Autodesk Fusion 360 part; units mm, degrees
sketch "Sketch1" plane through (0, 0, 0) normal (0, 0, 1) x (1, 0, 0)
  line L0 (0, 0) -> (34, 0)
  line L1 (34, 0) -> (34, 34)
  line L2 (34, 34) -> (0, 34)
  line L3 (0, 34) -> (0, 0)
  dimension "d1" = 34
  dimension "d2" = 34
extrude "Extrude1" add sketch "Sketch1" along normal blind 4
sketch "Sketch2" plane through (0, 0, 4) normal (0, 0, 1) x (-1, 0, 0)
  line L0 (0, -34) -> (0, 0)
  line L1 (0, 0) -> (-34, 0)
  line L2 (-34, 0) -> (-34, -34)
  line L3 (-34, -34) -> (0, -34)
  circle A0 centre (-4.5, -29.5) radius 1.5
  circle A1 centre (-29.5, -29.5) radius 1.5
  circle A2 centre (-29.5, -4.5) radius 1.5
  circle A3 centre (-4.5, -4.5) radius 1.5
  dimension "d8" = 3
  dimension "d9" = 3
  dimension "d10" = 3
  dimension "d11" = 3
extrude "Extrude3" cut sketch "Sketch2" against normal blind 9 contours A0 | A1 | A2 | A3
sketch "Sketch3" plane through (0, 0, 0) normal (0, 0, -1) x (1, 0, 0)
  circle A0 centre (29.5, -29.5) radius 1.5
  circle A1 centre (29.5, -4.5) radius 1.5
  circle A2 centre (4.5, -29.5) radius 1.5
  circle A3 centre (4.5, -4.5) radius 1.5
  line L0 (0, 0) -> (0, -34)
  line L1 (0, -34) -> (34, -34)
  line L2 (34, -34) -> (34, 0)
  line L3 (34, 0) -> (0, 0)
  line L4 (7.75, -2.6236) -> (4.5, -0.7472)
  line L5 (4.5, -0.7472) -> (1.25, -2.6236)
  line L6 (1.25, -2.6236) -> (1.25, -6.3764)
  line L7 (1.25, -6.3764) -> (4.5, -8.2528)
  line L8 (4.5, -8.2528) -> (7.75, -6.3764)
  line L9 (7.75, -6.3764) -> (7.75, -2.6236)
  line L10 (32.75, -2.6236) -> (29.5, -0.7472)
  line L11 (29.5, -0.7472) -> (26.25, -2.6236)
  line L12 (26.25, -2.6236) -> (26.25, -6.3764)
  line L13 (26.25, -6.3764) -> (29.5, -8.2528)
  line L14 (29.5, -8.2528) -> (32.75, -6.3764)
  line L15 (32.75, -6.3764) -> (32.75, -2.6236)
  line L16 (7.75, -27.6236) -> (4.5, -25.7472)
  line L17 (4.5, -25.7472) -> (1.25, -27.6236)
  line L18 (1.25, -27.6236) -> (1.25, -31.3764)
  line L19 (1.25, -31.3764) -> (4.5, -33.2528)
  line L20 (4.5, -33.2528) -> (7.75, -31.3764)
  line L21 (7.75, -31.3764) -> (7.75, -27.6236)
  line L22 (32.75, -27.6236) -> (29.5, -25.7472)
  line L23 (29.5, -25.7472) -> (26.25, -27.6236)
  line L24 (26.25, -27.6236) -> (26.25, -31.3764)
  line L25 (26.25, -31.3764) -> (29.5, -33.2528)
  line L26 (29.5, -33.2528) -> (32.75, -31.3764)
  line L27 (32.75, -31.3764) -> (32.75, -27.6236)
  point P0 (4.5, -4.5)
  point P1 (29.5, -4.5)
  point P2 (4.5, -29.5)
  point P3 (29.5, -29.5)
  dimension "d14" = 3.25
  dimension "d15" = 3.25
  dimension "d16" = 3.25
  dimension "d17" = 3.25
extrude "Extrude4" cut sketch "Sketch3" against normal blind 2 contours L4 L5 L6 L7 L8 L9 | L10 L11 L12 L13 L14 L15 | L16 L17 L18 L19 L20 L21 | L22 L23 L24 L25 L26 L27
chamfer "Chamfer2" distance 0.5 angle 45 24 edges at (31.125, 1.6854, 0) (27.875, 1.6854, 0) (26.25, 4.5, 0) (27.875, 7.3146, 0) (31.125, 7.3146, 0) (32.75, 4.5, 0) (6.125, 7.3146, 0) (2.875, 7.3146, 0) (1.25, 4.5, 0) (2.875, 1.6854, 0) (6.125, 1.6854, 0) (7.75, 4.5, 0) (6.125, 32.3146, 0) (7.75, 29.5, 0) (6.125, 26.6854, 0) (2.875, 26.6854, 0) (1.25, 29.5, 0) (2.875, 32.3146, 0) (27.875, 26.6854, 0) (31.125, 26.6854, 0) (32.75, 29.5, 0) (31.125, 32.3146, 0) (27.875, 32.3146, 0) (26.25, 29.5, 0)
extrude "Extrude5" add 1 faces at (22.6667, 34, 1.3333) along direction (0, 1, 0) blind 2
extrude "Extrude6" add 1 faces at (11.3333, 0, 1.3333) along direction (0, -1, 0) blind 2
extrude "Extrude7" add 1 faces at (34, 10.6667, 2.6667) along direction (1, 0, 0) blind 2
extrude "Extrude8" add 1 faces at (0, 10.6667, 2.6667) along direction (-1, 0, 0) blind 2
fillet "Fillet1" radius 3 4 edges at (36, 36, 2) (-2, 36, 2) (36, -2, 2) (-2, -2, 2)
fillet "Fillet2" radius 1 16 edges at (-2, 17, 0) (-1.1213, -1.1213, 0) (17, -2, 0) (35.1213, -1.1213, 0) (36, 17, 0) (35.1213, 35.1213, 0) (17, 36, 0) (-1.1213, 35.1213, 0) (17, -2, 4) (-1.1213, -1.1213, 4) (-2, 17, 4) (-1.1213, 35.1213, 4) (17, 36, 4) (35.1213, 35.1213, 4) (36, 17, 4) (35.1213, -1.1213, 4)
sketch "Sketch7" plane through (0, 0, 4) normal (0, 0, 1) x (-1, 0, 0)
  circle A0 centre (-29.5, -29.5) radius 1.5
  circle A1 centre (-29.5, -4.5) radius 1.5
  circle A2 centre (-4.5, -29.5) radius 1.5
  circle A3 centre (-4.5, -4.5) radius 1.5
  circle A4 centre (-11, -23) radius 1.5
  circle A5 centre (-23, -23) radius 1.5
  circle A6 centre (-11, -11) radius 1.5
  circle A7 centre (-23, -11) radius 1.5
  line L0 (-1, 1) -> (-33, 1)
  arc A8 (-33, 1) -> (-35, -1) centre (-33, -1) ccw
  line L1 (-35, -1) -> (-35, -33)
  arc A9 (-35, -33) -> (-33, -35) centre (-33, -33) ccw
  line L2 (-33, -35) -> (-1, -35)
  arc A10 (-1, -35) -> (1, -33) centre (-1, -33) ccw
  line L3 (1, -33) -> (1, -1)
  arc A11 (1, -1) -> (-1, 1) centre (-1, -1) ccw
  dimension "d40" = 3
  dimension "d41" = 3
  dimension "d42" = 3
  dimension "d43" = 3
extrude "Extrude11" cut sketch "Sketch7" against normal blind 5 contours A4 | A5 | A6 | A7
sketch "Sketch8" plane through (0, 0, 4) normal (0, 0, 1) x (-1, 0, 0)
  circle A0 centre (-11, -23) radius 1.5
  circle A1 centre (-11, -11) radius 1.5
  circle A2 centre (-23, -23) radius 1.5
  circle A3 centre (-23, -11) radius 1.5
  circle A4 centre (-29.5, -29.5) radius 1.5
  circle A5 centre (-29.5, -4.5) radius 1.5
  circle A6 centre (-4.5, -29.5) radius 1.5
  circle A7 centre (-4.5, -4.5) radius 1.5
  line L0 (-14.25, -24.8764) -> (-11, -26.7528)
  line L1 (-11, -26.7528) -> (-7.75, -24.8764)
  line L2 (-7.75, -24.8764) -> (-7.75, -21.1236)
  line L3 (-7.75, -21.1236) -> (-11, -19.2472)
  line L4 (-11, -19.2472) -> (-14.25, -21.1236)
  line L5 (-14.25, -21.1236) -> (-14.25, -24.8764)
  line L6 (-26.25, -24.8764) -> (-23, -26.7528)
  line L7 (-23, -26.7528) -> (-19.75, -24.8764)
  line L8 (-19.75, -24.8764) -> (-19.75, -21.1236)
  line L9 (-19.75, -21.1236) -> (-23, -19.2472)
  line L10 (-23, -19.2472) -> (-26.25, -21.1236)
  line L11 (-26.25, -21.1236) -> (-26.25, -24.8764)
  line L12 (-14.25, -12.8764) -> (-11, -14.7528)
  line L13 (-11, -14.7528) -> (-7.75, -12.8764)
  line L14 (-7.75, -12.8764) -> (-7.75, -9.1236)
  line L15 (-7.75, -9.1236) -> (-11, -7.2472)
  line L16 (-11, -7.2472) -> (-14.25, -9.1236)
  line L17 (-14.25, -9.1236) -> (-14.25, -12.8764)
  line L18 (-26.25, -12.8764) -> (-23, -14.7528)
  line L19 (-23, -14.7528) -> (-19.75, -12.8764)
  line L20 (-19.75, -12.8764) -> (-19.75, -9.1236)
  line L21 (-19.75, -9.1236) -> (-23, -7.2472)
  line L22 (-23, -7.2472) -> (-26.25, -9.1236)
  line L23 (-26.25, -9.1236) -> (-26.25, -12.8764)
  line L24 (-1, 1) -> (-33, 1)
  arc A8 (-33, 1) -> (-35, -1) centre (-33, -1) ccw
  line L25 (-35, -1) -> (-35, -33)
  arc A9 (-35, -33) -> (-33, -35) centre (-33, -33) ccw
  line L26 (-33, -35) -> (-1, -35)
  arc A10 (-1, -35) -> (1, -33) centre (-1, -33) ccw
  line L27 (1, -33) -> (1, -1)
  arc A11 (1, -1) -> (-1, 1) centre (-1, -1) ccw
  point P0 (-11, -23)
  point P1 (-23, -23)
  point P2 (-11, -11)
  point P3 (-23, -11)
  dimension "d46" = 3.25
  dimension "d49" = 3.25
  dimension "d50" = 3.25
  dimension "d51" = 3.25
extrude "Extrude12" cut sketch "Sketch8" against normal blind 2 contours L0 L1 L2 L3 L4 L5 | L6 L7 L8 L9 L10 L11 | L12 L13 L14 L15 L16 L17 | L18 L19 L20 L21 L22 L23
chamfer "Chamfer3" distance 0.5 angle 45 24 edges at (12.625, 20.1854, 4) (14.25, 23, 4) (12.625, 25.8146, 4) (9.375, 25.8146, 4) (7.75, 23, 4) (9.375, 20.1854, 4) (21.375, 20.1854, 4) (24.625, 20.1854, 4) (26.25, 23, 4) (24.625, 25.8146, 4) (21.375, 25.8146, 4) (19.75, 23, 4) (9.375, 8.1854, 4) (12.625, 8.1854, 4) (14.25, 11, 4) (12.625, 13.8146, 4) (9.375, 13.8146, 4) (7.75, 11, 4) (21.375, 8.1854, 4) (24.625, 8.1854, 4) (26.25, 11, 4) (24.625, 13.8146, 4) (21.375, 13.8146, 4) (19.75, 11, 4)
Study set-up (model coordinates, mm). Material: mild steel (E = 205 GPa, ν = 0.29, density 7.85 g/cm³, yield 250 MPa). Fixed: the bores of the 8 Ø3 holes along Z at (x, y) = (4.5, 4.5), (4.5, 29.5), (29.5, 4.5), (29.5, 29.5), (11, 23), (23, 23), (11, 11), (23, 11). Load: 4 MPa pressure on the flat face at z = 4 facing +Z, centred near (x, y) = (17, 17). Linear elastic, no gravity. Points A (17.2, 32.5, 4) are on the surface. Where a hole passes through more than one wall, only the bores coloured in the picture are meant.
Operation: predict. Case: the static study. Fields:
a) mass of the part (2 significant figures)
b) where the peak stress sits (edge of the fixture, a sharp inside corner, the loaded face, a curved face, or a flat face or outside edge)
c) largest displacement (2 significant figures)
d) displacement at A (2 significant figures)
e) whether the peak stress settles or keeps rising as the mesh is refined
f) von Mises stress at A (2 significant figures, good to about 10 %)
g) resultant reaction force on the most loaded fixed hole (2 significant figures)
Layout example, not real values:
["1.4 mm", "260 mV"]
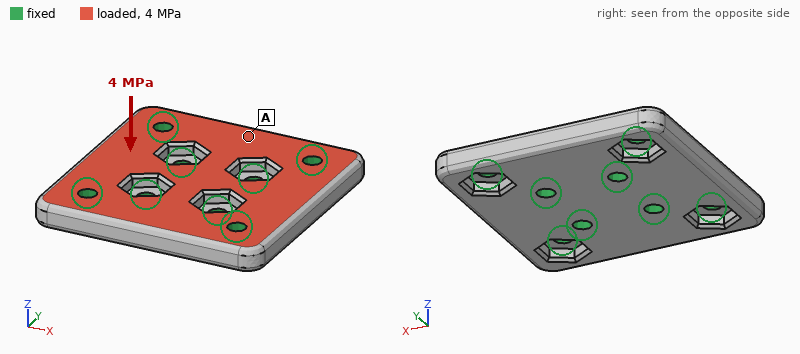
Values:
["39 g", "edge of the fixture", "5.3 µm", "4.0 µm", "keeps rising", "17 MPa", "640 N"]
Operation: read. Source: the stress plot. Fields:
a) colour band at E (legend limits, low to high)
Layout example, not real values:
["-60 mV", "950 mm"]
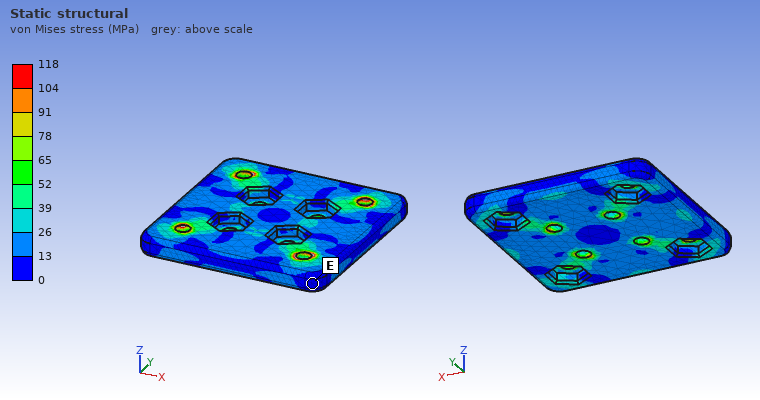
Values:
["0 to 13 MPa"]
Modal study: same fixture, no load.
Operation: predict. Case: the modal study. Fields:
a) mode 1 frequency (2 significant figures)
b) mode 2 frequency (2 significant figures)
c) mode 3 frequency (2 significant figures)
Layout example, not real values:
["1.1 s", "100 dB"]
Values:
["24 kHz", "26 kHz", "26 kHz"]
